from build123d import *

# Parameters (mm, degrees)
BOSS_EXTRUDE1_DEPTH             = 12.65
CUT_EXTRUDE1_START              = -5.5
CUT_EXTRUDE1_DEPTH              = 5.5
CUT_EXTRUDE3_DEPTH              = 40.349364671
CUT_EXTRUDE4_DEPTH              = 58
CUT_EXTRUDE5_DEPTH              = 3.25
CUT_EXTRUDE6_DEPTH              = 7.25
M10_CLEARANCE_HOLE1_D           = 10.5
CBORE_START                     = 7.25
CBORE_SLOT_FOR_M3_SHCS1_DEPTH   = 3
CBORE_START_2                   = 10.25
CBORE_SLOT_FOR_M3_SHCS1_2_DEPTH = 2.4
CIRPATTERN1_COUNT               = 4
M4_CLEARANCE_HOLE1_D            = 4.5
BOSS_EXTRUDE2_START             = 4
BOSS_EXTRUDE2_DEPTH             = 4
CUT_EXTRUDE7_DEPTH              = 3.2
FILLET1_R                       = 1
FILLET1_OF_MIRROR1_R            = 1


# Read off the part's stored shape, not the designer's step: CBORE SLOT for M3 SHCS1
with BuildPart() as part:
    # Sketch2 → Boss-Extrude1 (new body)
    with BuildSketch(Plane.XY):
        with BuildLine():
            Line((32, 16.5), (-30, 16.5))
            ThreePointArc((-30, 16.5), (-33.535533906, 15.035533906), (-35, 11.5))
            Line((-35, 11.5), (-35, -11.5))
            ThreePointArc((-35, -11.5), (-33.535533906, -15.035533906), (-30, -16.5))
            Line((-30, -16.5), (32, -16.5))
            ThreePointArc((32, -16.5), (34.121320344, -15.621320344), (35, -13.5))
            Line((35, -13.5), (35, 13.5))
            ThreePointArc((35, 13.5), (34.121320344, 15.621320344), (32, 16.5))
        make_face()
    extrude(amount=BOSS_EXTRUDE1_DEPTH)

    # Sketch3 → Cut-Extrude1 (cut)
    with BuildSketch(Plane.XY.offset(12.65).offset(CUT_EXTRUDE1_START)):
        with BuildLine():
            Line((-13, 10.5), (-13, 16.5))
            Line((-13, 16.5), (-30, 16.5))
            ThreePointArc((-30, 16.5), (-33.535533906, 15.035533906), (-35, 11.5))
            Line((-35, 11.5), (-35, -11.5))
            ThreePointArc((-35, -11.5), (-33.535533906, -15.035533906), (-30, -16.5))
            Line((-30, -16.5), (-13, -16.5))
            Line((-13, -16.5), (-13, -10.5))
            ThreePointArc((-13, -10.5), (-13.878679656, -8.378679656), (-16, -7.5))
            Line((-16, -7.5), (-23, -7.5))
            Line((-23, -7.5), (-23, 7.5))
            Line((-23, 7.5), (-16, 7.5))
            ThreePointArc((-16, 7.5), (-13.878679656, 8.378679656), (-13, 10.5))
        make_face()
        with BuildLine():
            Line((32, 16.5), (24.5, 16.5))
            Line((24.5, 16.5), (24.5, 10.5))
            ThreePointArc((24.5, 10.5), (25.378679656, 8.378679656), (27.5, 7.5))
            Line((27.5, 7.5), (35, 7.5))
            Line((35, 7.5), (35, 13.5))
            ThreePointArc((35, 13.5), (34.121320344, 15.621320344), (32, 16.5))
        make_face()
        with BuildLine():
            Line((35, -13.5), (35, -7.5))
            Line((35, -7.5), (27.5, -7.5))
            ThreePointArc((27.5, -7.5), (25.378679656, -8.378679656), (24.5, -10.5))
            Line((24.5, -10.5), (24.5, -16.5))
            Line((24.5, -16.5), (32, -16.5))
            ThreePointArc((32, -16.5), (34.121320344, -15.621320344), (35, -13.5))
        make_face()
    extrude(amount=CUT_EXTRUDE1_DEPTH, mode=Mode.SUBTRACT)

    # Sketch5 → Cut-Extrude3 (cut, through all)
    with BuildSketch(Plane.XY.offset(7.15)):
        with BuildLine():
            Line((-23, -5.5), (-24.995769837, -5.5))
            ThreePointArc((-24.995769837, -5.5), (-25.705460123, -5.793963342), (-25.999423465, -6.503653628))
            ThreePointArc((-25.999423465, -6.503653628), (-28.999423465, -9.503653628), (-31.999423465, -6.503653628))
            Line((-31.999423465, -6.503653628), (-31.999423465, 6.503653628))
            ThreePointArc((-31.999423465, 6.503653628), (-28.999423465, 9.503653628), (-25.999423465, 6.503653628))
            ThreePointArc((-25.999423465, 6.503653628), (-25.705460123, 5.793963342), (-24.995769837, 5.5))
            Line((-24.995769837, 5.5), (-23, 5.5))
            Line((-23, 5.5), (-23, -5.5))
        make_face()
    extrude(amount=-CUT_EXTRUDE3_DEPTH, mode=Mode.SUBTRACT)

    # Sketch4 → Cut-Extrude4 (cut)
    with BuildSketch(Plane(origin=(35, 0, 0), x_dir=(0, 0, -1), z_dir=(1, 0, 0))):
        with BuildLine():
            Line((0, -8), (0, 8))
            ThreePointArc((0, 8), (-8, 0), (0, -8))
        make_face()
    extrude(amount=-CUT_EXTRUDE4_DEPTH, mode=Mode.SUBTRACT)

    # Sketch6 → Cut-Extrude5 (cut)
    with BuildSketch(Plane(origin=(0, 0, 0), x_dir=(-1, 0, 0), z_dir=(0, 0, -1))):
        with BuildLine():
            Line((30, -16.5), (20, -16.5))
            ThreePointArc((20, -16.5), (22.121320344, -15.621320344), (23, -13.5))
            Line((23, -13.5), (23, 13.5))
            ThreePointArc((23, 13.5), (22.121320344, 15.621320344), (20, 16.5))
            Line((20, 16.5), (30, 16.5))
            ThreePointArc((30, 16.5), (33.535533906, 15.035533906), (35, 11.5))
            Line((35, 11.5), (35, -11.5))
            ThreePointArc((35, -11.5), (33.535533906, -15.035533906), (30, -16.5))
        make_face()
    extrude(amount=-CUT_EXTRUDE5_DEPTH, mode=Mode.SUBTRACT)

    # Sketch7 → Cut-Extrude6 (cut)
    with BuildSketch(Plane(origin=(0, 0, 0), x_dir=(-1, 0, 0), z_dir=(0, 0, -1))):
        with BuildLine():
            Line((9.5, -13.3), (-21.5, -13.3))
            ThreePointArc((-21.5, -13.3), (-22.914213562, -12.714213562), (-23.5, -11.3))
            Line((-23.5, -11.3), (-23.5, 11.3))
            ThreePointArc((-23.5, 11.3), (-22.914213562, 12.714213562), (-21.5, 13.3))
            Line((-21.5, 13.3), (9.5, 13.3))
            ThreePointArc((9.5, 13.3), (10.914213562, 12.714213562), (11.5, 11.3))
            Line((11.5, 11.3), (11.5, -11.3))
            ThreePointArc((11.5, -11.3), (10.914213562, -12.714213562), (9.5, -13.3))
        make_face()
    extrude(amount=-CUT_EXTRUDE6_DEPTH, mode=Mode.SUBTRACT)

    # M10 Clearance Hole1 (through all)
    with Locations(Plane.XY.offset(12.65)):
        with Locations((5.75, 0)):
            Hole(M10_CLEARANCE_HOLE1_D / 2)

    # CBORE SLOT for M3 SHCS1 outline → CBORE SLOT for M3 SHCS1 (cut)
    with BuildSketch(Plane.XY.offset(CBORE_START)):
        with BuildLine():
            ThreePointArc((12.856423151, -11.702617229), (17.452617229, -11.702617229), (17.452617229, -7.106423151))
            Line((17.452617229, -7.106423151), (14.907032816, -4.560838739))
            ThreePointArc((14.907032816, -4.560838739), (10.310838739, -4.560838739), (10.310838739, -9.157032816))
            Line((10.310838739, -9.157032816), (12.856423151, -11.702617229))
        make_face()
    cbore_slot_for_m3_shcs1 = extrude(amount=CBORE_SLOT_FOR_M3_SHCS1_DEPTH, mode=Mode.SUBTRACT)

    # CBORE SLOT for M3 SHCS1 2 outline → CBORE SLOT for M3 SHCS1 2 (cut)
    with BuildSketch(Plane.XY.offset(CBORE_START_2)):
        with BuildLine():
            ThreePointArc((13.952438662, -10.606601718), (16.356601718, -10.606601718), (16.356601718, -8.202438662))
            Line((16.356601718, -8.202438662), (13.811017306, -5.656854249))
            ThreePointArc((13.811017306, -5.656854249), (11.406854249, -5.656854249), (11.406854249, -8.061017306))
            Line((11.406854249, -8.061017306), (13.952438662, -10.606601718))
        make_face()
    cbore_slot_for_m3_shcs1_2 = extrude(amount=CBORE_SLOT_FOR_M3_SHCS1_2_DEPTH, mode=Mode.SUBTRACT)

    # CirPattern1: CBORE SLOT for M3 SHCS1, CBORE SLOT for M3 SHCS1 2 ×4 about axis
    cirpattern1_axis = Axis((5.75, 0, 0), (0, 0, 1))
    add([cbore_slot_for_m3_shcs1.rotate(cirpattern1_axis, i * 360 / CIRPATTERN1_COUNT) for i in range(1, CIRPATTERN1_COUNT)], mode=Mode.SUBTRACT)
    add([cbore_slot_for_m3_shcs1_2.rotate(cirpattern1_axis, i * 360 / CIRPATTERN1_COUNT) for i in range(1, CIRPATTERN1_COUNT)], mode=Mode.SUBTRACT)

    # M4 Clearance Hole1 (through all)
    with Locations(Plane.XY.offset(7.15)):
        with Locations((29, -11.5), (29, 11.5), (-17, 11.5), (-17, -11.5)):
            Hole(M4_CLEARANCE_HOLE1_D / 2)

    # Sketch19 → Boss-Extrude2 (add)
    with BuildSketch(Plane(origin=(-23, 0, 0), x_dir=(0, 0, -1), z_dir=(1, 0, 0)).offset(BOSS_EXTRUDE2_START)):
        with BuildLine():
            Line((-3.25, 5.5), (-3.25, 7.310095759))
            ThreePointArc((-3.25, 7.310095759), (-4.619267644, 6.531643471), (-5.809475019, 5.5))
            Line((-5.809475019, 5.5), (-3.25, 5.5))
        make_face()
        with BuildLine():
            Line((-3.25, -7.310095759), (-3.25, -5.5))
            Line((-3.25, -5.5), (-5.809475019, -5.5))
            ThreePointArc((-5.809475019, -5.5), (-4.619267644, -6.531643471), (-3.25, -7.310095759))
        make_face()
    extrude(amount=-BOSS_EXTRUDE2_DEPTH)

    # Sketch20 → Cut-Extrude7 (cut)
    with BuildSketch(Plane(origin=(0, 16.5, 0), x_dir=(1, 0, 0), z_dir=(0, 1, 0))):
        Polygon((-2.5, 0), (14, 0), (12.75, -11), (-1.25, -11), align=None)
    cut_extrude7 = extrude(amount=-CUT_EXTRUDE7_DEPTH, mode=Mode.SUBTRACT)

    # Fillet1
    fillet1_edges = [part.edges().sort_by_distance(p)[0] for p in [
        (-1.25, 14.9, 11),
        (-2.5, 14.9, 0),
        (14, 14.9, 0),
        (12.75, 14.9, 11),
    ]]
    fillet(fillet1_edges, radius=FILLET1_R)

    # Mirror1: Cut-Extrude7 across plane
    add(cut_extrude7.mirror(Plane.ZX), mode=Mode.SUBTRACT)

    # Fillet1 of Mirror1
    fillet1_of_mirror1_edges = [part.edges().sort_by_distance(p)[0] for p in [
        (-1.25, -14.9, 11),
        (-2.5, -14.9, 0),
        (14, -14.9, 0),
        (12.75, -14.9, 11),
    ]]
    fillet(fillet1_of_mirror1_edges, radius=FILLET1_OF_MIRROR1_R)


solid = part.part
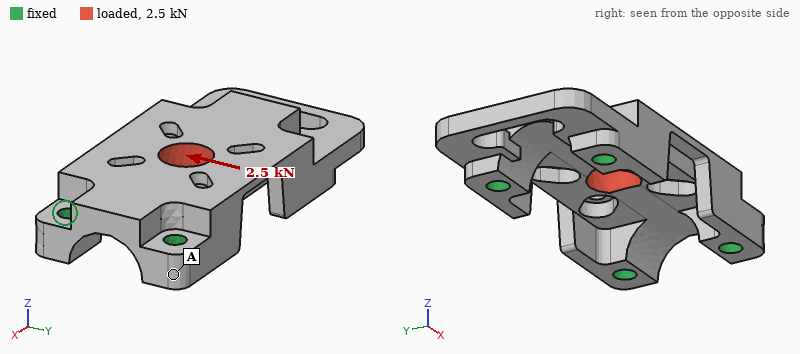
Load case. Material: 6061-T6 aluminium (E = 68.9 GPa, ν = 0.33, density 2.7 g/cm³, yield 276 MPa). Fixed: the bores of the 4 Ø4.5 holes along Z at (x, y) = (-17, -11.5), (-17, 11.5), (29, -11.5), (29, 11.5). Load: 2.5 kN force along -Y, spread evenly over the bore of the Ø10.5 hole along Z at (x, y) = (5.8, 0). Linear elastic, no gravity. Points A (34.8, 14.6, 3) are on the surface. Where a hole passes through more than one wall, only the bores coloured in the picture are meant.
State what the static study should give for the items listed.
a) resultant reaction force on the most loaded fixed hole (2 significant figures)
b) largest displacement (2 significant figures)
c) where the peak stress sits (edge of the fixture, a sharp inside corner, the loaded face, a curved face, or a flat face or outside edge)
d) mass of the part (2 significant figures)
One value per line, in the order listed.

830 N
18 µm
a curved face
30 g
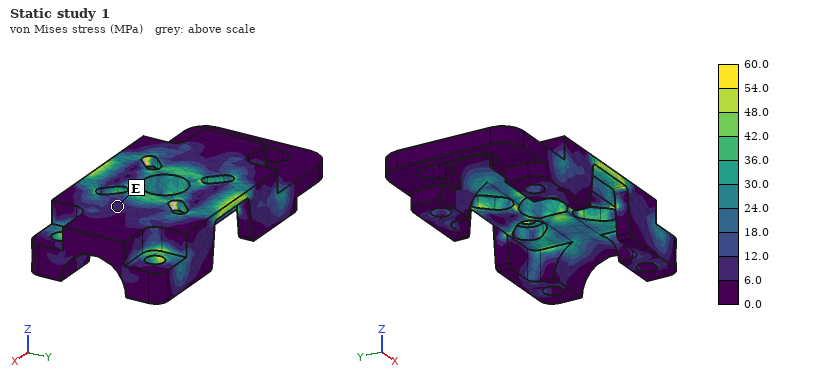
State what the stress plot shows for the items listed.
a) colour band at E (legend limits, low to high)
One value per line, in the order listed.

6.0 to 12.0 MPa
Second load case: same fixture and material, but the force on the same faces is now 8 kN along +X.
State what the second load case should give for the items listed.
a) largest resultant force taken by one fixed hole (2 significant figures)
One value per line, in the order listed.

2.1 kN
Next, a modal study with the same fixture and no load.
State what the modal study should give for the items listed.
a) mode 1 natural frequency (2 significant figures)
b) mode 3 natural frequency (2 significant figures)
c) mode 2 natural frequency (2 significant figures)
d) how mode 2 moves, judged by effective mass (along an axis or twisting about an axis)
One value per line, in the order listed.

12 kHz
19 kHz
16 kHz
along Z
